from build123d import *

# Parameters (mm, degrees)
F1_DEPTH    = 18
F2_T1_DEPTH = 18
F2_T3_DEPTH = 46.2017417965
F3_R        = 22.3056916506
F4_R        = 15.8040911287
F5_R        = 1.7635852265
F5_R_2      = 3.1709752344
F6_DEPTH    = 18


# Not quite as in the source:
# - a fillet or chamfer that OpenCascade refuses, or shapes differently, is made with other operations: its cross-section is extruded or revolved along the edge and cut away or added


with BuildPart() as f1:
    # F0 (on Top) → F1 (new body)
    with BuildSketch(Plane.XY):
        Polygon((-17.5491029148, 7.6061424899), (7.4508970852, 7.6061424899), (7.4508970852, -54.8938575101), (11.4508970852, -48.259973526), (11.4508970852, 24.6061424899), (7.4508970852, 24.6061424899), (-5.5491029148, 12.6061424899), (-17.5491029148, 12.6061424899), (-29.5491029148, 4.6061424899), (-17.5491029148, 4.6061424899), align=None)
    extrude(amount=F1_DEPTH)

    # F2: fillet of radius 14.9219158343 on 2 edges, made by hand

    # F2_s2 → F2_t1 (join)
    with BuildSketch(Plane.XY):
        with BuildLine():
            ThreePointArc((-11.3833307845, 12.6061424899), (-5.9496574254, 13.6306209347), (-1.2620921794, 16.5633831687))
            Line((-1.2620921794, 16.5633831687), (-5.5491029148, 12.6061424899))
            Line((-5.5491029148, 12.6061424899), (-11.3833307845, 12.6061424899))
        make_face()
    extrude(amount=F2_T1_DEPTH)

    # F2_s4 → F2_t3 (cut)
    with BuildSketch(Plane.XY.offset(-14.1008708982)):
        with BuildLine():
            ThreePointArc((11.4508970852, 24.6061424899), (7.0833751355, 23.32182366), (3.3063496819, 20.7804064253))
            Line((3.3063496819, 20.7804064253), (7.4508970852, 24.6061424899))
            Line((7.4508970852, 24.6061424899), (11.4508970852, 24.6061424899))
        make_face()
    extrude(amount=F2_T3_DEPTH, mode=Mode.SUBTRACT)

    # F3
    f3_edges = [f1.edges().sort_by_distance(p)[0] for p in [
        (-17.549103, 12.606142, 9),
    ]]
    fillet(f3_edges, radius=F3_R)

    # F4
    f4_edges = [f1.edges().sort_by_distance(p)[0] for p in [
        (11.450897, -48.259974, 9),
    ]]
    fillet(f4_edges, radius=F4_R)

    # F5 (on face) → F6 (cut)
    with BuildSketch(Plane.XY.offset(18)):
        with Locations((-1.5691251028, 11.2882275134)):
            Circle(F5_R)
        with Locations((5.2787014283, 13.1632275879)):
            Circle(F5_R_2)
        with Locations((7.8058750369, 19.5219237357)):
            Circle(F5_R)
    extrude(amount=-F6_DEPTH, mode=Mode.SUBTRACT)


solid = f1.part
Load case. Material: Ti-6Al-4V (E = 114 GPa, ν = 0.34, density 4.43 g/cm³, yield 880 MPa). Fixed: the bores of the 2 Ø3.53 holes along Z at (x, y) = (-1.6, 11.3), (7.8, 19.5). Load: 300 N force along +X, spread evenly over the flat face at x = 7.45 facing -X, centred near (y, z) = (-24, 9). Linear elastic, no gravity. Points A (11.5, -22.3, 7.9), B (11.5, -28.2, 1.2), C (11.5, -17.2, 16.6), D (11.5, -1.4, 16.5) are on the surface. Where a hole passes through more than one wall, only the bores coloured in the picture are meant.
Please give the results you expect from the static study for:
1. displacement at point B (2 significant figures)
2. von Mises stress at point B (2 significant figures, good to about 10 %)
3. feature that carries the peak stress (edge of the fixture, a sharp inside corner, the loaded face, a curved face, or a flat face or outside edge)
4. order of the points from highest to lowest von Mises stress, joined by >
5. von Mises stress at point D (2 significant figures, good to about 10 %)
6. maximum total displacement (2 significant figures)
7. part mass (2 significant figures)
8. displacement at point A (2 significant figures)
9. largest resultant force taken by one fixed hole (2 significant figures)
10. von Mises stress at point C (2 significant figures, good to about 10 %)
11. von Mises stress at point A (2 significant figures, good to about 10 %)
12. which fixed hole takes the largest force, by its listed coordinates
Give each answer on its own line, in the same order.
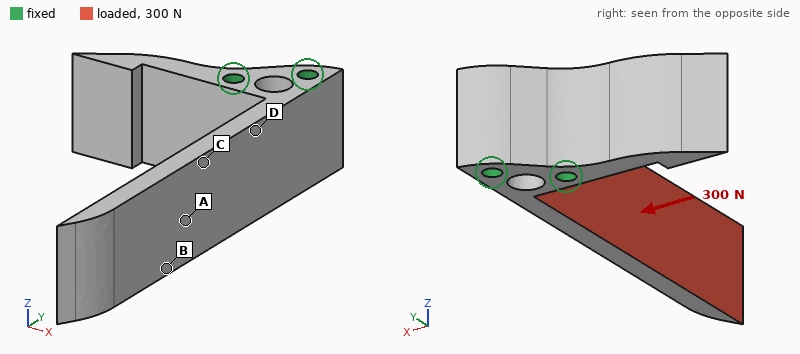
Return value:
0.46 mm
36 MPa
a flat face or outside edge
D > C > A > B
140 MPa
0.98 mm
40 g
0.35 mm
1.3 kN
72 MPa
54 MPa
(-1.6, 11.3)
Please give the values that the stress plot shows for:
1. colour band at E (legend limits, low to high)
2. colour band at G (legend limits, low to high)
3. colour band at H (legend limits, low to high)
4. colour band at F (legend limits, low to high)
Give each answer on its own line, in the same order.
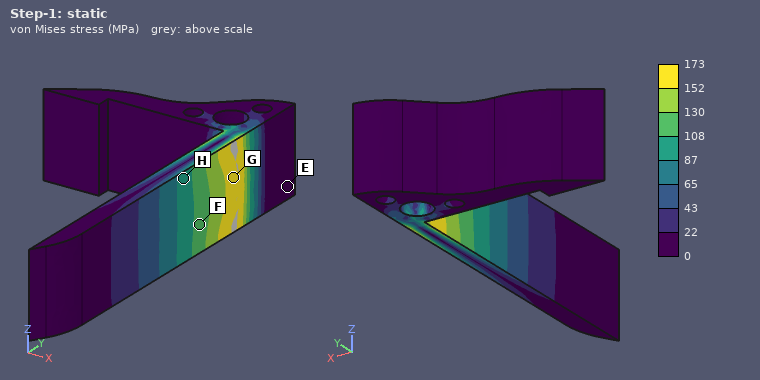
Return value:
0 to 22 MPa
152 to 173 MPa
87 to 108 MPa
108 to 130 MPa
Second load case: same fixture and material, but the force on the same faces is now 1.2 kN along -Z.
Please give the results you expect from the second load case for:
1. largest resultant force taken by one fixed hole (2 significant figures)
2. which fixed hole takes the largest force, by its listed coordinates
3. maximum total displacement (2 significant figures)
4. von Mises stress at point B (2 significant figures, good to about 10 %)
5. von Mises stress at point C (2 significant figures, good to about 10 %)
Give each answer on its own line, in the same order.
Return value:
1.5 kN
(-1.6, 11.3)
0.32 mm
25 MPa
51 MPa
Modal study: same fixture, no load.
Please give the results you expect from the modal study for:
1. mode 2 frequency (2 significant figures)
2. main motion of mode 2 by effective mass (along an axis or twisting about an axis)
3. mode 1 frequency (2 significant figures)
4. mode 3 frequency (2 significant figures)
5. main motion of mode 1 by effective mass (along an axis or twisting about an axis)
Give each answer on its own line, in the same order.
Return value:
3000 Hz
along Z
870 Hz
5300 Hz
along X
